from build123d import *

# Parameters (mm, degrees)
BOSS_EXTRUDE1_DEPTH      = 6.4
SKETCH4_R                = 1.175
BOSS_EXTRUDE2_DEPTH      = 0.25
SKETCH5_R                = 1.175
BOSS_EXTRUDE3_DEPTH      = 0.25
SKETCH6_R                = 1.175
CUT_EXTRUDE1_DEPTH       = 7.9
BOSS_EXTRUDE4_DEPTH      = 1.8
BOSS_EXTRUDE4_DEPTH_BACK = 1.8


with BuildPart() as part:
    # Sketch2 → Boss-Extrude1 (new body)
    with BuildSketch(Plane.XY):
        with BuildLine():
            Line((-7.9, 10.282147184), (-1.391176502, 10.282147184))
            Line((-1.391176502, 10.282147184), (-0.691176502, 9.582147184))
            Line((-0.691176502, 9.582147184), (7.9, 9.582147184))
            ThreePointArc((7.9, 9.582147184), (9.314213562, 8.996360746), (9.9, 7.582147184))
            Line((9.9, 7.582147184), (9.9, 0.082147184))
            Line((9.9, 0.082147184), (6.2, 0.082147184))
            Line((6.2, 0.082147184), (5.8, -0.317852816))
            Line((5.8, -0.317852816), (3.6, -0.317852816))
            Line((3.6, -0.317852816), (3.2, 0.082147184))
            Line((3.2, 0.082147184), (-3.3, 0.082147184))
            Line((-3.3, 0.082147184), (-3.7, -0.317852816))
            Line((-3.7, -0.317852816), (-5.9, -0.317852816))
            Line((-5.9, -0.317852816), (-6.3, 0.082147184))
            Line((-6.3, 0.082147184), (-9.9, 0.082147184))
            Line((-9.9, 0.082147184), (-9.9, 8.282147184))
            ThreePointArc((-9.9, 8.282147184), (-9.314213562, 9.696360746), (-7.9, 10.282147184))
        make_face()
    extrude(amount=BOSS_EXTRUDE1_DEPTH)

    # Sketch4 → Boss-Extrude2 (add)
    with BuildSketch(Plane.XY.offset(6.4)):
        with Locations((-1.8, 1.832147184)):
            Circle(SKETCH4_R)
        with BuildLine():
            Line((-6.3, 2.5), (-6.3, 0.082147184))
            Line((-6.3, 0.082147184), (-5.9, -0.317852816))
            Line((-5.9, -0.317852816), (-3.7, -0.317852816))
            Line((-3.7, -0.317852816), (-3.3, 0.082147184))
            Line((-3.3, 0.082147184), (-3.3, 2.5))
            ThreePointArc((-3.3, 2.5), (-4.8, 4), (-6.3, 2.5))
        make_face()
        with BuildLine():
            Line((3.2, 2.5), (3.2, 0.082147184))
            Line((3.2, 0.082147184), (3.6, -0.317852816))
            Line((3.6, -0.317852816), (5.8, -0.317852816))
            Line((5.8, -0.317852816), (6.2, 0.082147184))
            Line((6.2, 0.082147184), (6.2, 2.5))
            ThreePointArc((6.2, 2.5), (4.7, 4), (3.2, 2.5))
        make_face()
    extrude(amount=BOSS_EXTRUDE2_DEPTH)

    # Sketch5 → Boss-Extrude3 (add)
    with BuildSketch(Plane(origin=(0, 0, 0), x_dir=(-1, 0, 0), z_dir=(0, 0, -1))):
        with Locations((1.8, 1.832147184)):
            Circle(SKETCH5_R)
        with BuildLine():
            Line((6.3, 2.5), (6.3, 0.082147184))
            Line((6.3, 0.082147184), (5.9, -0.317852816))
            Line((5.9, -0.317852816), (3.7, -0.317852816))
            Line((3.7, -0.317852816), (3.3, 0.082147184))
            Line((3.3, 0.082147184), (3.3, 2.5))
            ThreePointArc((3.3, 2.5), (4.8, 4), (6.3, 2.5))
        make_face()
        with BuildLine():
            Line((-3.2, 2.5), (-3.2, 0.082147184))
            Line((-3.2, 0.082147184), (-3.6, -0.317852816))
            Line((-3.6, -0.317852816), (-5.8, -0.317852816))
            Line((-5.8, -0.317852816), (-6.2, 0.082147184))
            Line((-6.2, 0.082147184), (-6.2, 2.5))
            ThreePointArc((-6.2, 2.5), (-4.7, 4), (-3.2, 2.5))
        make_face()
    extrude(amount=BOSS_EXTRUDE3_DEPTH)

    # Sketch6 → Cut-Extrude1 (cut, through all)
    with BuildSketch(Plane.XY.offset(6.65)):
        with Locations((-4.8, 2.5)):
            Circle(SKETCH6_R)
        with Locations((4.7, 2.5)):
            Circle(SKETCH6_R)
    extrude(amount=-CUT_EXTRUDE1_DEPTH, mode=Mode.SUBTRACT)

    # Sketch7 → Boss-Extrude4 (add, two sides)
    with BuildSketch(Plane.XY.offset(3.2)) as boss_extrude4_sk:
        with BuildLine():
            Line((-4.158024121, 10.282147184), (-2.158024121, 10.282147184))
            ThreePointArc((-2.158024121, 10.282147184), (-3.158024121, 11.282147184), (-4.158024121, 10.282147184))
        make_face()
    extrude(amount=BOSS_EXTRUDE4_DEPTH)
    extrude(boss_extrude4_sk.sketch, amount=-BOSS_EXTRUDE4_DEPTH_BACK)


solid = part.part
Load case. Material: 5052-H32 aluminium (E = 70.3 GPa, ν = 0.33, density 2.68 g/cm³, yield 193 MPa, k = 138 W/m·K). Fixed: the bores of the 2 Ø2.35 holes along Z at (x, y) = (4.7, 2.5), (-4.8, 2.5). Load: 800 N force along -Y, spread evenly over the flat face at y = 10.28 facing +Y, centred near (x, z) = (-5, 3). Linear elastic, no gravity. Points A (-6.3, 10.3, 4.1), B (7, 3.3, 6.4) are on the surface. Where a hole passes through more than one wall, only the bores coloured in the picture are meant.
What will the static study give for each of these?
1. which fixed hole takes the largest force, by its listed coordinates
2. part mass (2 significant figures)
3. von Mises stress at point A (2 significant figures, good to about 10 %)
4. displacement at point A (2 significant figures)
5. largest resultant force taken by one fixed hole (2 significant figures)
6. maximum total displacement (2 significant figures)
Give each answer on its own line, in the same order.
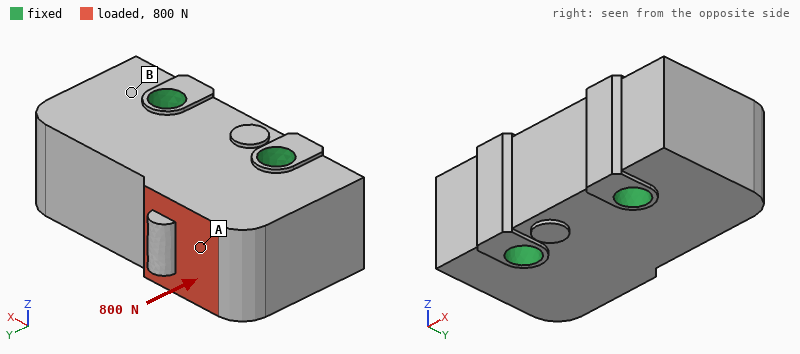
(-4.8, 2.5)
3.2 g
18 MPa
2.5 µm
760 N
2.6 µm
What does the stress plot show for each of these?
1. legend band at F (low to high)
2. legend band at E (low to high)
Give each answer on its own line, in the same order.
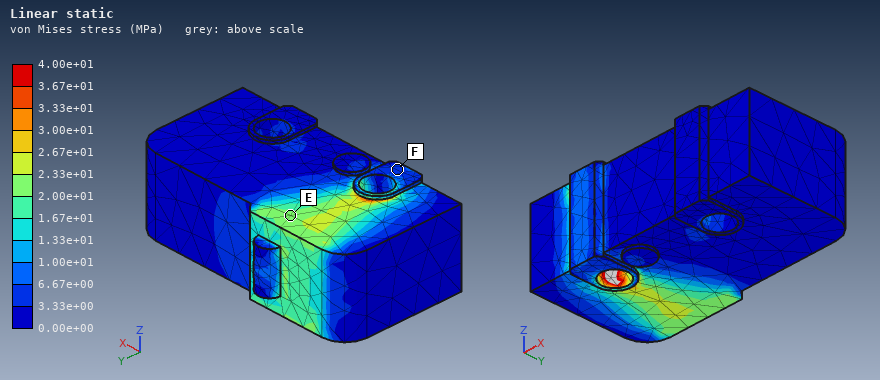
3.33e+00 to 6.67e+00 MPa
2.00e+01 to 2.33e+01 MPa
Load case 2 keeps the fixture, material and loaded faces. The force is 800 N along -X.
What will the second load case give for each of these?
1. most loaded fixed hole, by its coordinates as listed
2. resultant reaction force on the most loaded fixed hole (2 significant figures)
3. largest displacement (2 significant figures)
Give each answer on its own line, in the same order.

(4.7, 2.5)
680 N
6.6 µm
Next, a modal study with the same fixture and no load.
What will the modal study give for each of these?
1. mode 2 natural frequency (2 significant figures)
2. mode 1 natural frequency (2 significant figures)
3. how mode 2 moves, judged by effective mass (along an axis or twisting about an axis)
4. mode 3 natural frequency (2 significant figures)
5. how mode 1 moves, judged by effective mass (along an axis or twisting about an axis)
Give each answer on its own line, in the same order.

71 kHz
61 kHz
along X
75 kHz
along Z
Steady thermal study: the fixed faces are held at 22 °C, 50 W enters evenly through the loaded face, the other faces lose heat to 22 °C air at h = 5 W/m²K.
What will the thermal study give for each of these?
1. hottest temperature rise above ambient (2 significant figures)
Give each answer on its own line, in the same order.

48 K
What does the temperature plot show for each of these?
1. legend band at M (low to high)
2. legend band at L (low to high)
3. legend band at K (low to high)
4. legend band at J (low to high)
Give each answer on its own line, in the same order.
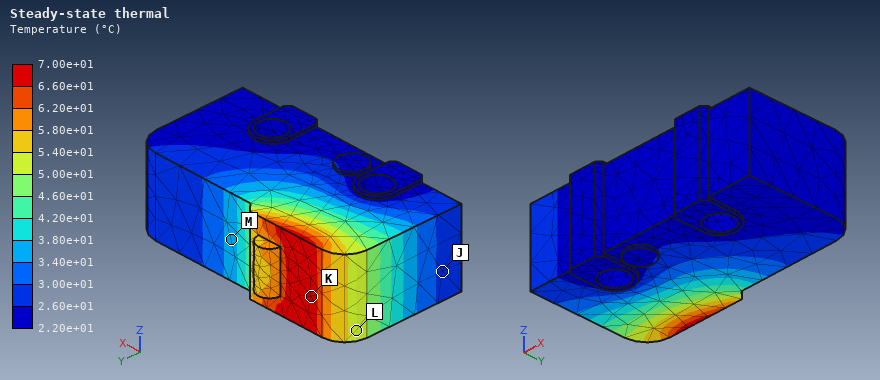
3.40e+01 to 3.80e+01 °C
5.00e+01 to 5.40e+01 °C
6.60e+01 to 7.00e+01 °C
2.60e+01 to 3.00e+01 °C
